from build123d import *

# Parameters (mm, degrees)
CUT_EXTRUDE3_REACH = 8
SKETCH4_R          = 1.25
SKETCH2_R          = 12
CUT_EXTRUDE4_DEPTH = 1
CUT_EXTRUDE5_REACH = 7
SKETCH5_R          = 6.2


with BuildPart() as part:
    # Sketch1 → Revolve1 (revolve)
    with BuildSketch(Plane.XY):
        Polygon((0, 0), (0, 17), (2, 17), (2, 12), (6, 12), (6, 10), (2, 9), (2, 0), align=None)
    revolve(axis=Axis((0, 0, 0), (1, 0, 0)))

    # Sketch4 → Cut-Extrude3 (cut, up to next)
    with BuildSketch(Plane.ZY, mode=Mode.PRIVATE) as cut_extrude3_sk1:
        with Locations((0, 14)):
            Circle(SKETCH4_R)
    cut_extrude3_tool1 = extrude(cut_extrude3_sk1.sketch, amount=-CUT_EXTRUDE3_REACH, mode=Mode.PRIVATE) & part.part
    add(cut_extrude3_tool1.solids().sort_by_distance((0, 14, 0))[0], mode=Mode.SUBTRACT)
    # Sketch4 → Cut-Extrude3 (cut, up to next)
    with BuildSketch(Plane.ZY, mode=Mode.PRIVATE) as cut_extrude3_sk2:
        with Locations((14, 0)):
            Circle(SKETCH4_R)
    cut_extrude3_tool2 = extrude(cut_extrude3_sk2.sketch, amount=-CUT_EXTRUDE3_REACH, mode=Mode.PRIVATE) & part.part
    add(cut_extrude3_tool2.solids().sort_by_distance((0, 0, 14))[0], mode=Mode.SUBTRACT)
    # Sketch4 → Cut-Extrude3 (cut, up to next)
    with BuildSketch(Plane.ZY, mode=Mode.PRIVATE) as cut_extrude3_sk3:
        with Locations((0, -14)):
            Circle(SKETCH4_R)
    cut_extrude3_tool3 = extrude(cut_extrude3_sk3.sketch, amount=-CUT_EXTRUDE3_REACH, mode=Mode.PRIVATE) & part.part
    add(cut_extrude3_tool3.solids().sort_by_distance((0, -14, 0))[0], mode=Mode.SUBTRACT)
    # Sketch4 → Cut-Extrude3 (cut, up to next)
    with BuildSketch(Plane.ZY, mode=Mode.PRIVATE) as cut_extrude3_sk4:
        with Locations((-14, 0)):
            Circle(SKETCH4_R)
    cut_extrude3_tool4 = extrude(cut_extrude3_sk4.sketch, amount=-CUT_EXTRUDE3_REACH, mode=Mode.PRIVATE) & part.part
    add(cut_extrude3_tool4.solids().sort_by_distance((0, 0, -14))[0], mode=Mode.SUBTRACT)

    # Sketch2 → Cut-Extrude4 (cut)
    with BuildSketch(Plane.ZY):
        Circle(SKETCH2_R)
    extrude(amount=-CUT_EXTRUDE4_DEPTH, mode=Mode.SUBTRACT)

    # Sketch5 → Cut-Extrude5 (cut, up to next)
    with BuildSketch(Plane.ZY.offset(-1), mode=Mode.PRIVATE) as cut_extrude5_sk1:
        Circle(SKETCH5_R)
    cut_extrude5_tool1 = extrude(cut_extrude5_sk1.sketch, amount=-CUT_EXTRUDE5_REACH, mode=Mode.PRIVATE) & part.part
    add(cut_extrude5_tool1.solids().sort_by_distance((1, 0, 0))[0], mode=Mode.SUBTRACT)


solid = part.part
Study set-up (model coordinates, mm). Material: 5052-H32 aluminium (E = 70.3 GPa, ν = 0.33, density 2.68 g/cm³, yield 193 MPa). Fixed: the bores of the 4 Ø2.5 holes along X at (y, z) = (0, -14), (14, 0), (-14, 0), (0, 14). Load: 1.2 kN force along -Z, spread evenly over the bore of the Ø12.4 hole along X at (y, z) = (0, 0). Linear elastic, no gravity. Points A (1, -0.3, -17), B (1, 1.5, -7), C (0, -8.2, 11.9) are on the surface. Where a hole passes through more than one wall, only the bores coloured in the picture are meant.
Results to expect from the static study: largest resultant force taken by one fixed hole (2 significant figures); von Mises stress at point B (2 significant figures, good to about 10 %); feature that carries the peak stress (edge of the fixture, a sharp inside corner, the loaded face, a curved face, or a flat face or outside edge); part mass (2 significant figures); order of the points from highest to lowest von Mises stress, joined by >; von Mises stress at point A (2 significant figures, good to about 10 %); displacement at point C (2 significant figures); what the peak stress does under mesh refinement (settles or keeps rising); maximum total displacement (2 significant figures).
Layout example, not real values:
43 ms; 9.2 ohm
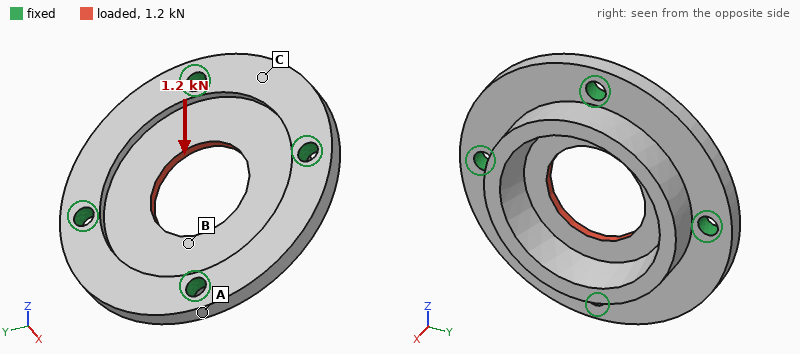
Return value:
320 N; 36 MPa; edge of the fixture; 5.0 g; B > A > C; 16 MPa; 2.1 µm; keeps rising; 5.3 µm
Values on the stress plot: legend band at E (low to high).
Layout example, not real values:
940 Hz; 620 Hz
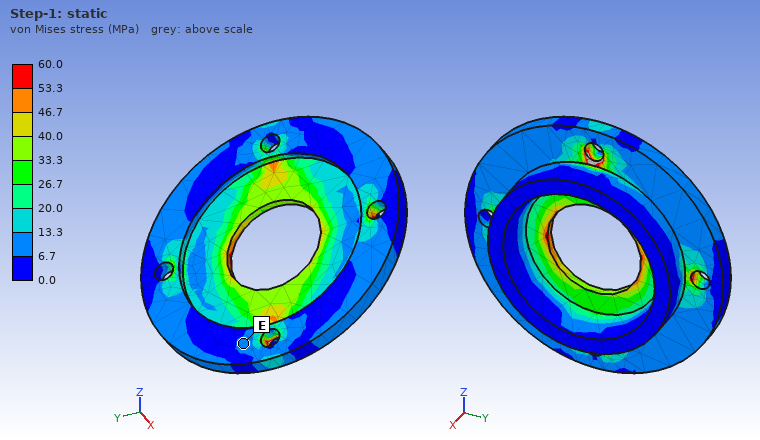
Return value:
6.7 to 13.3 MPa
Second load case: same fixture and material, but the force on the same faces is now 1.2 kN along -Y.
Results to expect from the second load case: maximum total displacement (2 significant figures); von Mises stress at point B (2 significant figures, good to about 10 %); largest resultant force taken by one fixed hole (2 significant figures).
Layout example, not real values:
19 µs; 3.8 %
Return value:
5.2 µm; 29 MPa; 320 N
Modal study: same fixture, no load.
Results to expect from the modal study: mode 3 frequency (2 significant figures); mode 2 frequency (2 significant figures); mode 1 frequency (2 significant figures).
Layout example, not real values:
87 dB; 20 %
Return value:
27 kHz; 27 kHz; 23 kHz
